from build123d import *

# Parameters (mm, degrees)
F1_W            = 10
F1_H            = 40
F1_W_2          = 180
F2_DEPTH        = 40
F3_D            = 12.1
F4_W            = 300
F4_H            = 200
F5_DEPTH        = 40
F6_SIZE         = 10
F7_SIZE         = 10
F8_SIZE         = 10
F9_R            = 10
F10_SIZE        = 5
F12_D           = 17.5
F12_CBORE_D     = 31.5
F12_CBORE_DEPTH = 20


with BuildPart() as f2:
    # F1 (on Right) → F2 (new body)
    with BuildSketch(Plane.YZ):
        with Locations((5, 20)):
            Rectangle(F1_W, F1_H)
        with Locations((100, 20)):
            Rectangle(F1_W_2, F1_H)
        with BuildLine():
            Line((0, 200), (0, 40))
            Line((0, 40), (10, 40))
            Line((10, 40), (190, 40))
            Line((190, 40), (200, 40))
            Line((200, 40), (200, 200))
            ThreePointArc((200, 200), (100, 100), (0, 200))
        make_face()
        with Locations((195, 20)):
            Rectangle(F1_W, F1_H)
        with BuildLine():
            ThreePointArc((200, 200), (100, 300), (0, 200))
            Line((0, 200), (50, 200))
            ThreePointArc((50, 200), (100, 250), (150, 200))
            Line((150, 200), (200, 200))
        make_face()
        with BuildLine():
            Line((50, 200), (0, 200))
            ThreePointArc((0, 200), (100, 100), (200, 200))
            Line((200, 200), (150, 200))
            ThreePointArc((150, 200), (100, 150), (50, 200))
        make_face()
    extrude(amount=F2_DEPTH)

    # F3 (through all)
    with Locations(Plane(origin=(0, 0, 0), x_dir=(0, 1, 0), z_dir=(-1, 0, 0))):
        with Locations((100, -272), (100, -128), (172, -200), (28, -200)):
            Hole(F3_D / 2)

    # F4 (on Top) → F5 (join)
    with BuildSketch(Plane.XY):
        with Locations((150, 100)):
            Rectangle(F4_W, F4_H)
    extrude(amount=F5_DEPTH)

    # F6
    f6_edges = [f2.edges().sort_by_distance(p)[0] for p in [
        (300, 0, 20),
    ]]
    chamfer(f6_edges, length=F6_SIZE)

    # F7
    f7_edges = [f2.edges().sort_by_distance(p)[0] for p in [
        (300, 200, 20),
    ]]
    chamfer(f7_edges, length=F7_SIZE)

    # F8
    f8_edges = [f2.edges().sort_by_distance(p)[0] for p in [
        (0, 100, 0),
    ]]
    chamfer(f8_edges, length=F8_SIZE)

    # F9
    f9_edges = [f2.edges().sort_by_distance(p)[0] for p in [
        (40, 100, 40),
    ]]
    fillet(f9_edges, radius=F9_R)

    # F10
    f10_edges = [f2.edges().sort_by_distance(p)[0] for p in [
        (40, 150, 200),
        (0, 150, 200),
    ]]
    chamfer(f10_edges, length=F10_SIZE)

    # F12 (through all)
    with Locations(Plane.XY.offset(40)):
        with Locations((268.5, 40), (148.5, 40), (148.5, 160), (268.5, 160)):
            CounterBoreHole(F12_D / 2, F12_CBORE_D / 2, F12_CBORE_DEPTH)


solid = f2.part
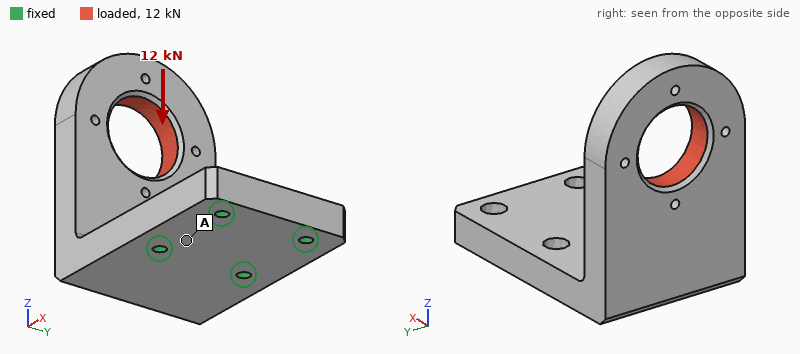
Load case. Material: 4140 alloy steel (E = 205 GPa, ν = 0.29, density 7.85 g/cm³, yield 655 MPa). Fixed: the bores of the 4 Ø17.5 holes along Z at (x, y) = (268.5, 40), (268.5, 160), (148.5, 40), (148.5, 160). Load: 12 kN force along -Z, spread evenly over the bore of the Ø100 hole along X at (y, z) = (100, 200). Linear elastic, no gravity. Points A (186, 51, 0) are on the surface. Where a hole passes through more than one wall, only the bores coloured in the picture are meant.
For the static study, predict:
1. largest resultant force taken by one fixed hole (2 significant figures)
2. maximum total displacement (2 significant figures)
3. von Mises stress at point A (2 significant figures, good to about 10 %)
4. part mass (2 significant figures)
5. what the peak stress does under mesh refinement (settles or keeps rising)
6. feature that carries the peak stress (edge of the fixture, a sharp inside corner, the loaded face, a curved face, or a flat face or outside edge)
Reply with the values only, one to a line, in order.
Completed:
13 kN
0.20 mm
6.7 MPa
30 kg
keeps rising
edge of the fixture
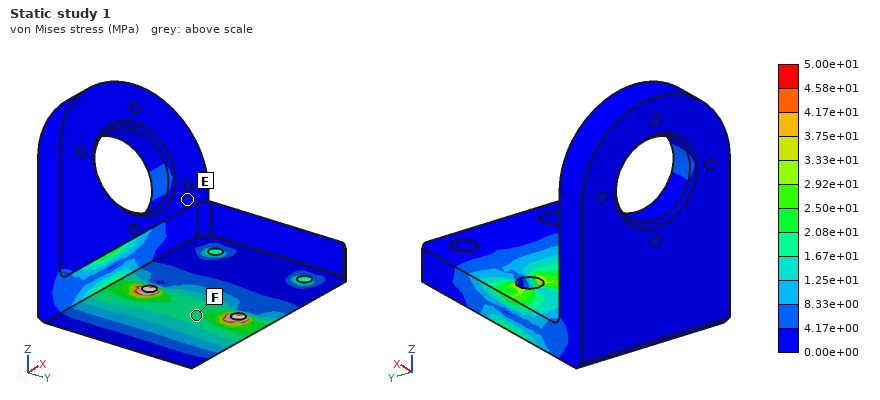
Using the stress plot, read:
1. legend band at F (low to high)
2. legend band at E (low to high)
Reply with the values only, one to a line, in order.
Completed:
1.67e+01 to 2.08e+01 MPa
0.00e+00 to 4.17e+00 MPa
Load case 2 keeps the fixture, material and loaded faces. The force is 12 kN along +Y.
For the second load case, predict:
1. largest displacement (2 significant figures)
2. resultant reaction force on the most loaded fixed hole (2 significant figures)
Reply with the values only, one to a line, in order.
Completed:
0.18 mm
24 kN
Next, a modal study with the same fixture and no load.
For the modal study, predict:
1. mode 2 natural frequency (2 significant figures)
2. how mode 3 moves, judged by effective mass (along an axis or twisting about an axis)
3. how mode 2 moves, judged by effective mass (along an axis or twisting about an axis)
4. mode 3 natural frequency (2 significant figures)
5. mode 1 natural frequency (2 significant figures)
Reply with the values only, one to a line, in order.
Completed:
510 Hz
along Z
along Y
850 Hz
280 Hz
